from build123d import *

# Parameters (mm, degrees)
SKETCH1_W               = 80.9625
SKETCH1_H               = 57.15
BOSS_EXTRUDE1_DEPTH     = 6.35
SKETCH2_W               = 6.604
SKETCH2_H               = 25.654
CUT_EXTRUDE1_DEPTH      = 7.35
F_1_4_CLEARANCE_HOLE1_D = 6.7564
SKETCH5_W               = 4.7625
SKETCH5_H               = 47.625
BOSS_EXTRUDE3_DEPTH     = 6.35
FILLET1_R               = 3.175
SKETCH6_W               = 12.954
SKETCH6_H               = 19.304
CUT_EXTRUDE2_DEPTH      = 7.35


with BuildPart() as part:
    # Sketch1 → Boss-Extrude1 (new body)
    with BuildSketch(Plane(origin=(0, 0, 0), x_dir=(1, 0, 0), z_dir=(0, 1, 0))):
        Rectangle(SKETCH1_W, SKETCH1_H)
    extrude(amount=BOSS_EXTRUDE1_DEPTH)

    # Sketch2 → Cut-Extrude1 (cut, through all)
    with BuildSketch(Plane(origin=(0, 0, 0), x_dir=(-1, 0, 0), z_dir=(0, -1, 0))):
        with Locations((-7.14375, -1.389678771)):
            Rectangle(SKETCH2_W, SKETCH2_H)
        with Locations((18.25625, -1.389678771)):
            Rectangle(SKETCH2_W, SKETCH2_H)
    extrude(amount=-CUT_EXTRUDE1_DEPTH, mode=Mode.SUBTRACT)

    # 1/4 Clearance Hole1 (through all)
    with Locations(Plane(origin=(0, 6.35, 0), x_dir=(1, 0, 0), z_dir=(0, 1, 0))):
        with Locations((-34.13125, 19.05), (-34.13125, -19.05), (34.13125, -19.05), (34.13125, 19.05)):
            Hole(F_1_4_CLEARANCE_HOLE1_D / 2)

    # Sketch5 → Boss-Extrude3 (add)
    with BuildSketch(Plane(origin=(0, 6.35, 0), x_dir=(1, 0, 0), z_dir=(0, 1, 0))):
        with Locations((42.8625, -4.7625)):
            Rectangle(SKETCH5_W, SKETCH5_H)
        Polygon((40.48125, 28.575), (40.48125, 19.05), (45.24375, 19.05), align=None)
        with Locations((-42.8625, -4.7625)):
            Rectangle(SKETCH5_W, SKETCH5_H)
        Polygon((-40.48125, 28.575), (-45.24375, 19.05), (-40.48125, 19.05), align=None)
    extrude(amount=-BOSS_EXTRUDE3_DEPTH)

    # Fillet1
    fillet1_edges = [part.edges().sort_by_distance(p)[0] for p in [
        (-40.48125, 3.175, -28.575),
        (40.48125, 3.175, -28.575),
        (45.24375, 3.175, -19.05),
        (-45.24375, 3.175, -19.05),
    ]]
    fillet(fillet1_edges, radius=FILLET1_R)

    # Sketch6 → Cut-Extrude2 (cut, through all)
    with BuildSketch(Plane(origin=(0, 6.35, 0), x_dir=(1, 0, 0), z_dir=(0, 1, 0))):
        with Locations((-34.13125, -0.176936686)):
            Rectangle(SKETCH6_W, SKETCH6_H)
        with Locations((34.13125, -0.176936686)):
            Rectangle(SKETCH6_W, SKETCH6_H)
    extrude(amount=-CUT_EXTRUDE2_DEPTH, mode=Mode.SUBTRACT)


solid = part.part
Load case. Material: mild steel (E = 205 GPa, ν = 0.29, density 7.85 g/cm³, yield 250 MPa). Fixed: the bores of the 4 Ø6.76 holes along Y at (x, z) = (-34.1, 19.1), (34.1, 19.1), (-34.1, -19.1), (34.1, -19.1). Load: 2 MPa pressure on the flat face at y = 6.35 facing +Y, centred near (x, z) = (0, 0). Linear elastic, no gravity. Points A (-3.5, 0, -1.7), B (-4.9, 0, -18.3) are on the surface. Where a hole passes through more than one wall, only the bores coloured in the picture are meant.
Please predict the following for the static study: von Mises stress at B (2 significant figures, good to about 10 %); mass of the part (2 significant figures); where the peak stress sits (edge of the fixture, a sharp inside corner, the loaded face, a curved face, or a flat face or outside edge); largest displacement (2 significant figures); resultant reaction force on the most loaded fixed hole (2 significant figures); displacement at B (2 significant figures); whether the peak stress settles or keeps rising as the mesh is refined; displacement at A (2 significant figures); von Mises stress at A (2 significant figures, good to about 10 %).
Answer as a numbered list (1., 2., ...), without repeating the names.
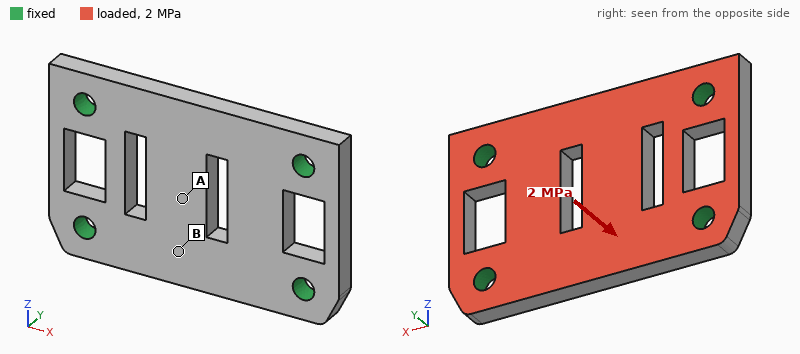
1. 56 MPa
2. 210 g
3. edge of the fixture
4. 40 µm
5. 2.1 kN
6. 30 µm
7. keeps rising
8. 35 µm
9. 27 MPa
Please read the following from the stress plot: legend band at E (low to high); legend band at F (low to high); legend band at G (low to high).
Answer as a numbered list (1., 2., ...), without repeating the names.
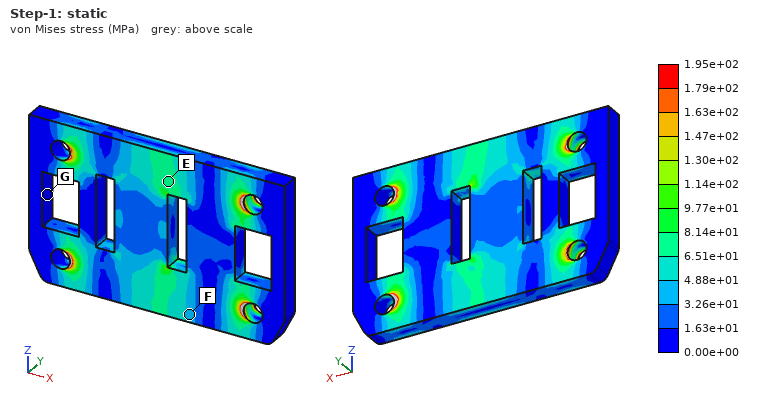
1. 6.51e+01 to 8.14e+01 MPa
2. 3.26e+01 to 4.88e+01 MPa
3. 0.00e+00 to 1.63e+01 MPa
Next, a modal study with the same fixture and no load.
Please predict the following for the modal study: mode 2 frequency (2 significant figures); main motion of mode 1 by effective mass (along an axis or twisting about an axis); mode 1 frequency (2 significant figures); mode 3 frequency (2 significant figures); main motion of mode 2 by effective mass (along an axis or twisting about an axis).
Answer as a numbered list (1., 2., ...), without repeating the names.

1. 8600 Hz
2. along Y
3. 6200 Hz
4. 14 kHz
5. twisting about X
